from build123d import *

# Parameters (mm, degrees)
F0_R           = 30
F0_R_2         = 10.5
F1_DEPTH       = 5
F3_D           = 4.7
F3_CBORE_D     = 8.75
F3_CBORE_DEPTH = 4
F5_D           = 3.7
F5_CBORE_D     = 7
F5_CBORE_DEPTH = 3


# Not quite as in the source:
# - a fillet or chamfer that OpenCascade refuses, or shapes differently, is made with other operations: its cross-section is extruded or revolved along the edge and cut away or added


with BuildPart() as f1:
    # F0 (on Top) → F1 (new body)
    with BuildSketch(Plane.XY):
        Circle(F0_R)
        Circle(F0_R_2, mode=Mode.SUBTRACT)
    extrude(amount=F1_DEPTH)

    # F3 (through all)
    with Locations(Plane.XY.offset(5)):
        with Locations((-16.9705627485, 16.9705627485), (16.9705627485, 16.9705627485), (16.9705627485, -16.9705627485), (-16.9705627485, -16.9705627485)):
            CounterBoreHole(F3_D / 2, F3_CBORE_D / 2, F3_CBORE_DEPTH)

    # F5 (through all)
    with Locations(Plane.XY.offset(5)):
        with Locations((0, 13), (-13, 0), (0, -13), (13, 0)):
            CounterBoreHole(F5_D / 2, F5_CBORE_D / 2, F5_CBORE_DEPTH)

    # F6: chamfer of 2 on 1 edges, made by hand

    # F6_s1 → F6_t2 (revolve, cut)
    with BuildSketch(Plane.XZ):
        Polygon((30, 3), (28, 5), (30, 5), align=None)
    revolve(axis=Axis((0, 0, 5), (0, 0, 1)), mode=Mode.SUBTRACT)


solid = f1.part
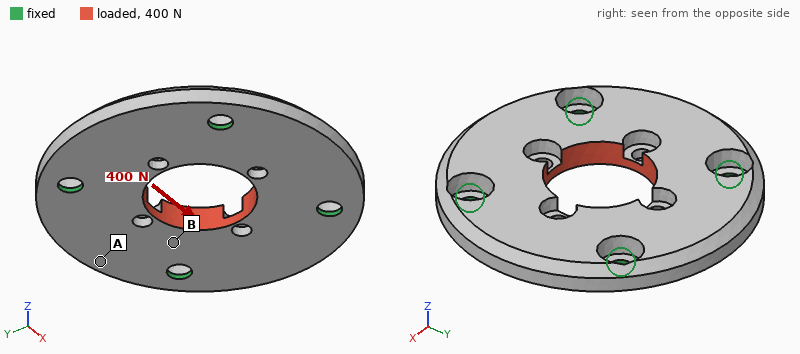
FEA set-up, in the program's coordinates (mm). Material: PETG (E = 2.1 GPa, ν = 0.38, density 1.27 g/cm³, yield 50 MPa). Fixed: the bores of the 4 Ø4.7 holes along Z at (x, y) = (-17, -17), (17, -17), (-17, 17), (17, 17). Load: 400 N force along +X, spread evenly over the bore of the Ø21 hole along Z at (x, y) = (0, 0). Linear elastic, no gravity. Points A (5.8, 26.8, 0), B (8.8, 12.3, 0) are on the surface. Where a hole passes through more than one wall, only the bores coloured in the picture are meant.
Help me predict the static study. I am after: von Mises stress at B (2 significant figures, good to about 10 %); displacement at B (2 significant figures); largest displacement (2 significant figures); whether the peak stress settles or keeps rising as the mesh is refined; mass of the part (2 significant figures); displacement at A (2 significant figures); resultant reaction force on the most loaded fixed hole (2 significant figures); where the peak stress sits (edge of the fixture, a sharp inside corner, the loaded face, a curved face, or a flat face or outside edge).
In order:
2.4 MPa
21 µm
50 µm
keeps rising
13 g
13 µm
100 N
edge of the fixture
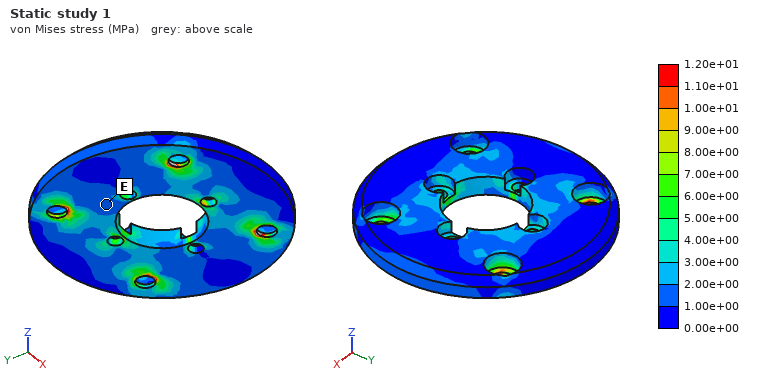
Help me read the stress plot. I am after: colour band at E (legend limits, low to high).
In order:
1.00e+00 to 2.00e+00 MPa
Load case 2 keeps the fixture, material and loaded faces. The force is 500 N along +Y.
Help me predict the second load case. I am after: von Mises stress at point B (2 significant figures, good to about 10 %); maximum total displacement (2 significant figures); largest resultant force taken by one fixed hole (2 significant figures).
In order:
1.9 MPa
62 µm
130 N
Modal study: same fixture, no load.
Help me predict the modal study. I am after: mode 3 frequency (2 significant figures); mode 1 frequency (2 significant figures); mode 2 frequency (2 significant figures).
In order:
2700 Hz
2100 Hz
2700 Hz
